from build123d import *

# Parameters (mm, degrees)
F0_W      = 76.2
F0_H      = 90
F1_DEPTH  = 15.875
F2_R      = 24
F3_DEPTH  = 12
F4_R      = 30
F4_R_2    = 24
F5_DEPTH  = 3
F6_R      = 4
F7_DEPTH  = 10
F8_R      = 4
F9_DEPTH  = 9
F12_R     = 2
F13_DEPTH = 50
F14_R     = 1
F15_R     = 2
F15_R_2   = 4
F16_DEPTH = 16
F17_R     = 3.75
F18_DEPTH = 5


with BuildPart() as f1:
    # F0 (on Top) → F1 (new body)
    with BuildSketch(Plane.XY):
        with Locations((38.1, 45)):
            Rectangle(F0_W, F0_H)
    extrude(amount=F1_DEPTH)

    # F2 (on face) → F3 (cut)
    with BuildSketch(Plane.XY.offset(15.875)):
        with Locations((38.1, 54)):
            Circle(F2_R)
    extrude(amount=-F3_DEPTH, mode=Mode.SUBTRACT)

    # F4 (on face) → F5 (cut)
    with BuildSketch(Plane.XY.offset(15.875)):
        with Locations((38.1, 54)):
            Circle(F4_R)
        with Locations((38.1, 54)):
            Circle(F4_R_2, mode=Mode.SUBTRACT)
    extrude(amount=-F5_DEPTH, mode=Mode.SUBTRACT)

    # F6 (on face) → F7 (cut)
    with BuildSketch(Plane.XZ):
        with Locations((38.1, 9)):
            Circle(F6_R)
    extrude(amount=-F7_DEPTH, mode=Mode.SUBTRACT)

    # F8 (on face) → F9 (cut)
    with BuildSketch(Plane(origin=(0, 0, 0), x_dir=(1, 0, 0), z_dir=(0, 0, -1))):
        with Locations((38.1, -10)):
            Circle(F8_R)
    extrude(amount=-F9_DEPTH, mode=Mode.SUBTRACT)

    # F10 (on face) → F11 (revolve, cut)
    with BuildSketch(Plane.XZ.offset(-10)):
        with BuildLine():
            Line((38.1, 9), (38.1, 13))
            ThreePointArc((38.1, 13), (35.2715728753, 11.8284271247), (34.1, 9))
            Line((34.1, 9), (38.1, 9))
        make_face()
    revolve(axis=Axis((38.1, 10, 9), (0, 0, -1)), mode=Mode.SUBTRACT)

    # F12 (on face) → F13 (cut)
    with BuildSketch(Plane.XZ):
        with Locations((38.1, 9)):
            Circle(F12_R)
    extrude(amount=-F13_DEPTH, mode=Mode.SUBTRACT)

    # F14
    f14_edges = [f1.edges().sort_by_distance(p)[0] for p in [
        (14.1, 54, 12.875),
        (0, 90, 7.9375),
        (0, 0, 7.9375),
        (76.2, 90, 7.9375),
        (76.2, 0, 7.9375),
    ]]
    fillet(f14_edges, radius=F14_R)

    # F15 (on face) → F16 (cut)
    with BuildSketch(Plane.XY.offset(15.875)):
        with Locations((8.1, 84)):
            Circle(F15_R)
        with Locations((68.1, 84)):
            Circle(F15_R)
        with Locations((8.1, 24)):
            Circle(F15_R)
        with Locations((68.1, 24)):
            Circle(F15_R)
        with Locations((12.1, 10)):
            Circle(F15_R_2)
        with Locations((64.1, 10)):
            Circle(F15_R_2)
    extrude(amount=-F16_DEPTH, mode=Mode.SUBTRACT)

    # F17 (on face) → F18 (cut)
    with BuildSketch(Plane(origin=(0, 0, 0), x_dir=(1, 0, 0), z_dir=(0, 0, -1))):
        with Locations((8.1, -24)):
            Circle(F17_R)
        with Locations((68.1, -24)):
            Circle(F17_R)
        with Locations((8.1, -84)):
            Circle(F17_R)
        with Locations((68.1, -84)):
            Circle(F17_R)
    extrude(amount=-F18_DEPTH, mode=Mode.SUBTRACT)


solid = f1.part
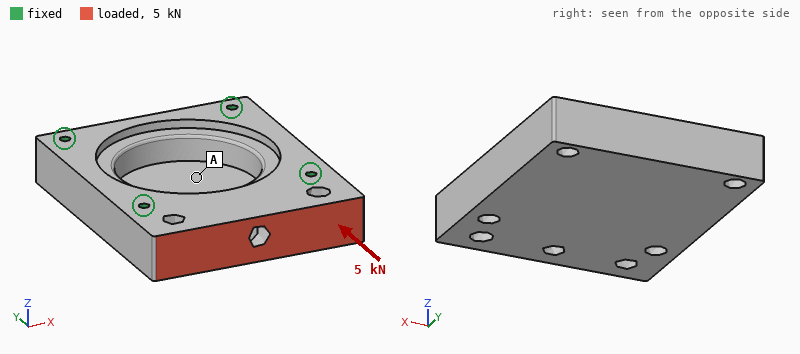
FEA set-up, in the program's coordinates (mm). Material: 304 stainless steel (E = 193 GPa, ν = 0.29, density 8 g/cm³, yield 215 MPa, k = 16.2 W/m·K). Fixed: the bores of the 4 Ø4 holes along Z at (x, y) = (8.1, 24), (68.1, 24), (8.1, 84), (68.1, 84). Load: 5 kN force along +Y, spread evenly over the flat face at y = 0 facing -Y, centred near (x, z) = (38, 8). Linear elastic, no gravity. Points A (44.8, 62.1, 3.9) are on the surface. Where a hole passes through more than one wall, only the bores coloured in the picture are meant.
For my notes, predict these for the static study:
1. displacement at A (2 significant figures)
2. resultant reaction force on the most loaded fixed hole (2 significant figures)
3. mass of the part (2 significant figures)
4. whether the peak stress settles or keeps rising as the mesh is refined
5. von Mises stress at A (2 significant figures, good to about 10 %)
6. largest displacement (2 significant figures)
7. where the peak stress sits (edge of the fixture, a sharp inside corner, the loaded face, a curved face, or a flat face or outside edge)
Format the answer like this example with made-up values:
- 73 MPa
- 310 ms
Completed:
- 0.46 µm
- 2.1 kN
- 640 g
- keeps rising
- 3.1 MPa
- 1.9 µm
- edge of the fixture
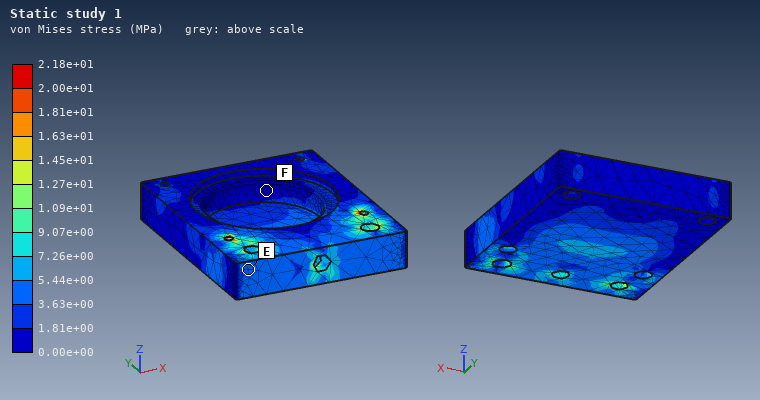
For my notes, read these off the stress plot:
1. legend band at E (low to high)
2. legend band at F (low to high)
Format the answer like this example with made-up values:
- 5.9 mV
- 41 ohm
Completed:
- 3.63e+00 to 5.44e+00 MPa
- 0.00e+00 to 1.81e+00 MPa
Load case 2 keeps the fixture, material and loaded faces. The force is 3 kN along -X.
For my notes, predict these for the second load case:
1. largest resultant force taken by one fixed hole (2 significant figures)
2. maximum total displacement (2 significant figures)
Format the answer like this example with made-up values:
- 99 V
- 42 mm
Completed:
- 1.8 kN
- 2.4 µm
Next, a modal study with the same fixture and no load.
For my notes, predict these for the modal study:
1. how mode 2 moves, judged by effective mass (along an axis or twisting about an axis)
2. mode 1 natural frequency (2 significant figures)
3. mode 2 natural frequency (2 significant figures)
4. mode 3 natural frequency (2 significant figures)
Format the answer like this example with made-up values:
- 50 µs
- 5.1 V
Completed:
- along Z
- 8600 Hz
- 10 kHz
- 13 kHz
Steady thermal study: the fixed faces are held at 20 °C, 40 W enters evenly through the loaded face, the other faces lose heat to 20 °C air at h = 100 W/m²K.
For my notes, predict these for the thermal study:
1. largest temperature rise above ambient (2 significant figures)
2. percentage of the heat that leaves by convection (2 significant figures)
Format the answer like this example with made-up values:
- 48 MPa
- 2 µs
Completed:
- 57 K
- 57 %
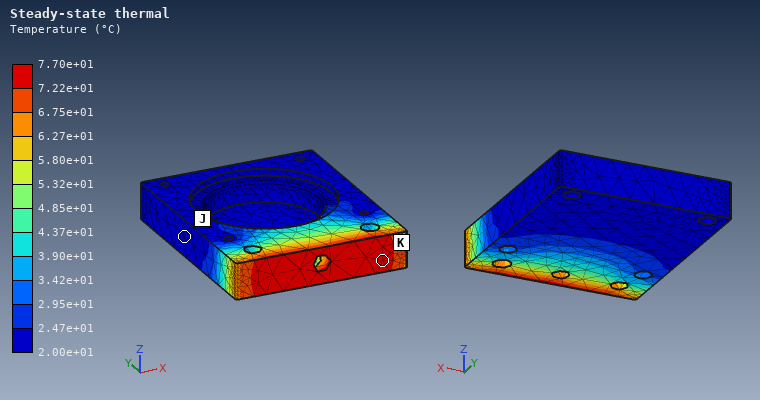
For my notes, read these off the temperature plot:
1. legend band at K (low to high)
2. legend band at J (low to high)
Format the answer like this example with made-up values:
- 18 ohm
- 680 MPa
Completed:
- 7.22e+01 to 7.70e+01 °C
- 2.00e+01 to 2.47e+01 °C
